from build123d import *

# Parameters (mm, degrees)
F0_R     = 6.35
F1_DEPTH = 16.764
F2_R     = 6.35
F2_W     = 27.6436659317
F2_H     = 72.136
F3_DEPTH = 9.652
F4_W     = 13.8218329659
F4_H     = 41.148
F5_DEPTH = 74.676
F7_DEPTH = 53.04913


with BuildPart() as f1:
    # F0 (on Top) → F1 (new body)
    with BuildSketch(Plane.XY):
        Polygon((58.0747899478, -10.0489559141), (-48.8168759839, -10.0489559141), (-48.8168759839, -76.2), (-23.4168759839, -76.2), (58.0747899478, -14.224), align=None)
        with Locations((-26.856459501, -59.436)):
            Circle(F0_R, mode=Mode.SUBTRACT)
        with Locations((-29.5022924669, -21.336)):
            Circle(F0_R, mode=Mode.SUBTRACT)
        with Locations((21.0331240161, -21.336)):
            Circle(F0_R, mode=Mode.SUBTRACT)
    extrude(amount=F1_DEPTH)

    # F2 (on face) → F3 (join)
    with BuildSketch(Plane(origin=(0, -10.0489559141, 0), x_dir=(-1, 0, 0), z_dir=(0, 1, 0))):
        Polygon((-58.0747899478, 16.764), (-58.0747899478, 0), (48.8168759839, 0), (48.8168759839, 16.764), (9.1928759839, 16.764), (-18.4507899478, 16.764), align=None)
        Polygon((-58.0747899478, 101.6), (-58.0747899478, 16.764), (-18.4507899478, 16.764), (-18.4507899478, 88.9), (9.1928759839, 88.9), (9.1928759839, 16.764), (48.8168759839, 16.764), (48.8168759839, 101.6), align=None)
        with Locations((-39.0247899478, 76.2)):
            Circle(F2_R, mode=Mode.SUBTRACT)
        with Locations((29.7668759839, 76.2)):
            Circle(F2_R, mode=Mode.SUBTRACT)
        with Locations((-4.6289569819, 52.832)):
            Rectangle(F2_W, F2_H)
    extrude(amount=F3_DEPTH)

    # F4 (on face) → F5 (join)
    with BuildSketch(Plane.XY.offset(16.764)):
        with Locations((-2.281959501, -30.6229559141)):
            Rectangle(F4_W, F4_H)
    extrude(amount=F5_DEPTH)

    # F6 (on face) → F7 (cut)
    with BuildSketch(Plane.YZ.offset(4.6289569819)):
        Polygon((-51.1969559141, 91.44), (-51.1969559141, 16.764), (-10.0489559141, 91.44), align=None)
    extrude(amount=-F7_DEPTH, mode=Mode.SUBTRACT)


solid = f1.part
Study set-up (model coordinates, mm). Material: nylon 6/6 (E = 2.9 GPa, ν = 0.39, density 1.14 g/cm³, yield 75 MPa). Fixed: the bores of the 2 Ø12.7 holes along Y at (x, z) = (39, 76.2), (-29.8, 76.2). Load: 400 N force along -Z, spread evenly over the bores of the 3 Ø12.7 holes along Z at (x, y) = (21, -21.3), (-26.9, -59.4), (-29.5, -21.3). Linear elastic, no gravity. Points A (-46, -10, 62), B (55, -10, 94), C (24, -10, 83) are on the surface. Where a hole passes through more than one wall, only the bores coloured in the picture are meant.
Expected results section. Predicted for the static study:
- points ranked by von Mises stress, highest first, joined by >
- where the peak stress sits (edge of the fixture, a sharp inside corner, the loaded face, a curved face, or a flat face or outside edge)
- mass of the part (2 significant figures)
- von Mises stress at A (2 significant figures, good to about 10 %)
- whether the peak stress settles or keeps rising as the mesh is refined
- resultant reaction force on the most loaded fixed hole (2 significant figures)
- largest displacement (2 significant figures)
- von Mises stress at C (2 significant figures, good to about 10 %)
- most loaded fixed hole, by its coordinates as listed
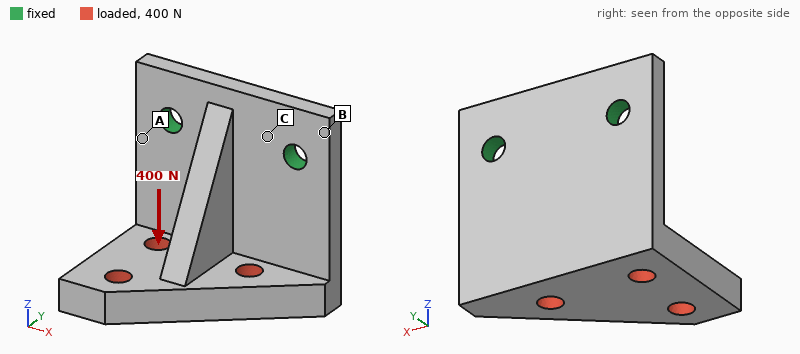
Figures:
A > C > B
edge of the fixture
220 g
4.2 MPa
keeps rising
300 N
0.86 mm
2.2 MPa
(-29.8, 76.2)
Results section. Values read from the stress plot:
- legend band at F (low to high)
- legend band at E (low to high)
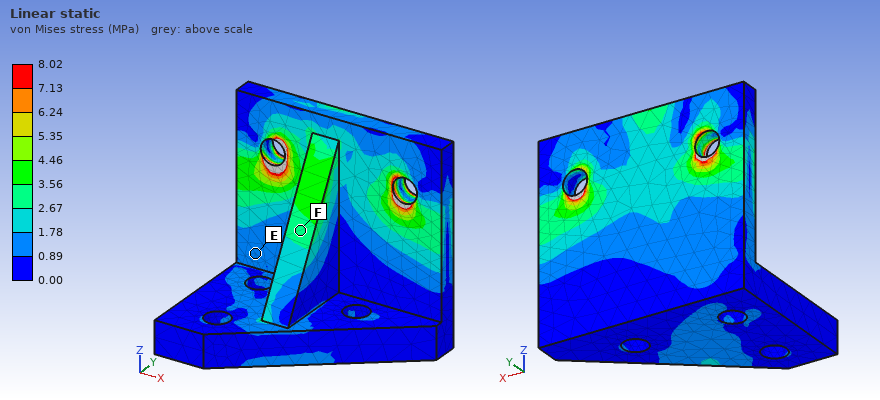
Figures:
2.67 to 3.56 MPa
0.89 to 1.78 MPa
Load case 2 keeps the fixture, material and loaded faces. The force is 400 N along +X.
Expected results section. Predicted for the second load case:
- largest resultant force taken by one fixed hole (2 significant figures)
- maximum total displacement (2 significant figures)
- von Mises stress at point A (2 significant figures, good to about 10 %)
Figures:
450 N
0.53 mm
2.0 MPa
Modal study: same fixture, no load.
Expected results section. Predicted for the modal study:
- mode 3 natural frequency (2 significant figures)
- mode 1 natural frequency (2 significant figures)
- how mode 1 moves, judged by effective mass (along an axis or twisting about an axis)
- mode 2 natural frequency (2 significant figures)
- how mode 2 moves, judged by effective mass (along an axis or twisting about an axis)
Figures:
1200 Hz
260 Hz
along Y
490 Hz
along X
